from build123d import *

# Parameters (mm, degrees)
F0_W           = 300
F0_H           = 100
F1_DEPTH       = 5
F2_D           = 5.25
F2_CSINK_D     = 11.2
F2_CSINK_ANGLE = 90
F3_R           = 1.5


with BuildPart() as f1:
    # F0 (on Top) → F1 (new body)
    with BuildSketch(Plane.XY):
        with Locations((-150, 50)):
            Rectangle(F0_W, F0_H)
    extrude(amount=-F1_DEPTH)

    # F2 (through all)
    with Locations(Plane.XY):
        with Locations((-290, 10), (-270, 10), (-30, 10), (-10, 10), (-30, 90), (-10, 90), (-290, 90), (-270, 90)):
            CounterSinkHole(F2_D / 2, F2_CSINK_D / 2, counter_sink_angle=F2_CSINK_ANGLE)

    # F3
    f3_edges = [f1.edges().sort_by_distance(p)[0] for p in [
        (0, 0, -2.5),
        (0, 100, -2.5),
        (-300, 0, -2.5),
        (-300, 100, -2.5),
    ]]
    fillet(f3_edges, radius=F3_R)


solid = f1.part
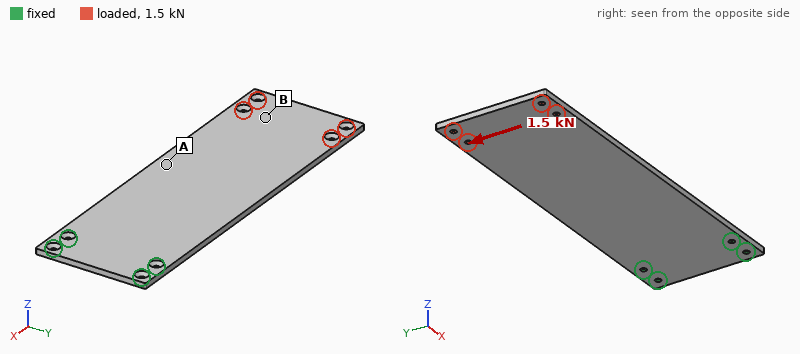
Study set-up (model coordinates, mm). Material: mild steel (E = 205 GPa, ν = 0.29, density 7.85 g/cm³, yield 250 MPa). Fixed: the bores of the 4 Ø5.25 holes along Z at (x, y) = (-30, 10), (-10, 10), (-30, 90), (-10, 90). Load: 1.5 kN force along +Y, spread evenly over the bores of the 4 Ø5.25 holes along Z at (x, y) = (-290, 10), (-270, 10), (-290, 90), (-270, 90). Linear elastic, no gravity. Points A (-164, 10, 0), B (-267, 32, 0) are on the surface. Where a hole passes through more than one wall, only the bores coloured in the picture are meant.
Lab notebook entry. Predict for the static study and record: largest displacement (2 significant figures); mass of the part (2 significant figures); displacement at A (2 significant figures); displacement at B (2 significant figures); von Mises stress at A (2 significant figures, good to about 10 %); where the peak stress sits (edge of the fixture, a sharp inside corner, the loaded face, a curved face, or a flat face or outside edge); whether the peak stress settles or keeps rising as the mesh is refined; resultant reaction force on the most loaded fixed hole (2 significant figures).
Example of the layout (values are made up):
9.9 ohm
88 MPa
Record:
0.16 mm
1.2 kg
0.064 mm
0.11 mm
17 MPa
edge of the fixture
keeps rising
3.5 kN
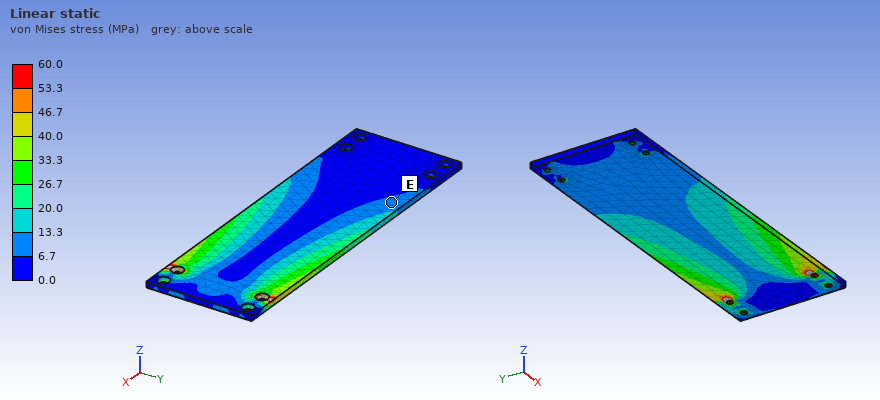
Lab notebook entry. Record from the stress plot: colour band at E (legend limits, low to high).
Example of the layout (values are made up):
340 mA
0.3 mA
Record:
6.7 to 13.3 MPa
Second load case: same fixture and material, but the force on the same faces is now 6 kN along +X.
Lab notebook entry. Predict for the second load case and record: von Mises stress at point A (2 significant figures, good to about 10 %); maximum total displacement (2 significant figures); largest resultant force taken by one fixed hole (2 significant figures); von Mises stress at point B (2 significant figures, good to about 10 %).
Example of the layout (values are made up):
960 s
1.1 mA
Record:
9.5 MPa
1.5 mm
2.2 kN
12 MPa
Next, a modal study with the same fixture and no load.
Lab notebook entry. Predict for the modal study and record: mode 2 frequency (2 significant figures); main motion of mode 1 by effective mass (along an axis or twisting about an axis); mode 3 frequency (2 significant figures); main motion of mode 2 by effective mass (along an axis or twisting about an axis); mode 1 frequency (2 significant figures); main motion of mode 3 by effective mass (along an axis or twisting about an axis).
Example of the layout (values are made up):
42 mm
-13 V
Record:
320 Hz
along Z
340 Hz
twisting about X
54 Hz
along Z
